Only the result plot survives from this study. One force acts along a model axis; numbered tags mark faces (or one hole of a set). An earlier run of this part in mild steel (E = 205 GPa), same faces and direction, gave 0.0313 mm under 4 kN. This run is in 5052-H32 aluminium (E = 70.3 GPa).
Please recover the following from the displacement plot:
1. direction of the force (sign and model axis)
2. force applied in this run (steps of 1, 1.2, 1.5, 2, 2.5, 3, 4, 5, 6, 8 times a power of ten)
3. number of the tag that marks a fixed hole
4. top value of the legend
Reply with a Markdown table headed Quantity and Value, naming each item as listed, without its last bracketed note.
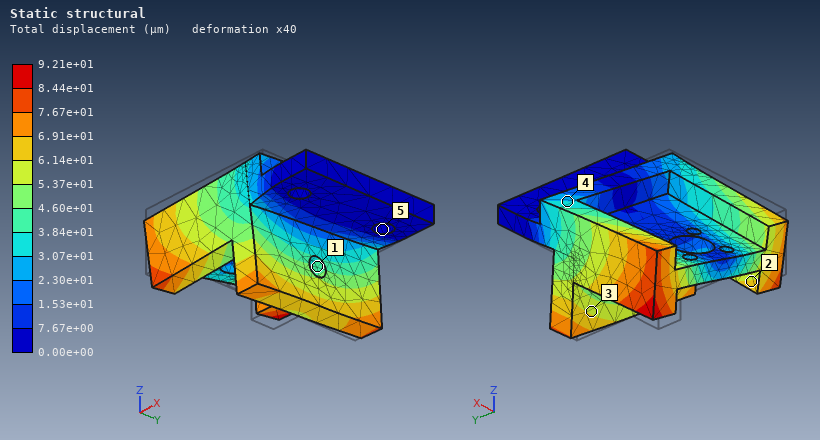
| Quantity | Value |
|---|---|
| direction of the force | +Y |
| force applied in this run | 4 kN |
| number of the tag that marks a fixed hole | 5 |
| top value of the legend | 9.21e+01 µm |
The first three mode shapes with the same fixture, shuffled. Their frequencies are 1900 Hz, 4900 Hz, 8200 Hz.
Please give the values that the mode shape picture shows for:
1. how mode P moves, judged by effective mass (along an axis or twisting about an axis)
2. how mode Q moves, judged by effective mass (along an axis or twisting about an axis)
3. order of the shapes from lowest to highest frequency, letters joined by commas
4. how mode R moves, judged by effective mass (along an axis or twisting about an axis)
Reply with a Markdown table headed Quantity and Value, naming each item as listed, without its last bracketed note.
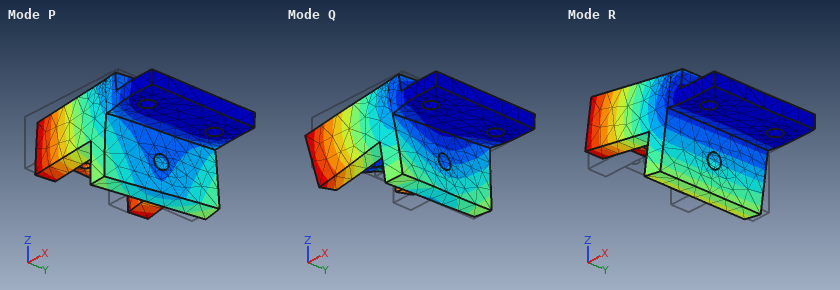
| Quantity | Value |
|---|---|
| how mode P moves, judged by effective mass | along Y |
| how mode Q moves, judged by effective mass | twisting about X |
| order of the shapes from lowest to highest frequency, letters joined by commas | R, Q, P |
| how mode R moves, judged by effective mass | along Z |
